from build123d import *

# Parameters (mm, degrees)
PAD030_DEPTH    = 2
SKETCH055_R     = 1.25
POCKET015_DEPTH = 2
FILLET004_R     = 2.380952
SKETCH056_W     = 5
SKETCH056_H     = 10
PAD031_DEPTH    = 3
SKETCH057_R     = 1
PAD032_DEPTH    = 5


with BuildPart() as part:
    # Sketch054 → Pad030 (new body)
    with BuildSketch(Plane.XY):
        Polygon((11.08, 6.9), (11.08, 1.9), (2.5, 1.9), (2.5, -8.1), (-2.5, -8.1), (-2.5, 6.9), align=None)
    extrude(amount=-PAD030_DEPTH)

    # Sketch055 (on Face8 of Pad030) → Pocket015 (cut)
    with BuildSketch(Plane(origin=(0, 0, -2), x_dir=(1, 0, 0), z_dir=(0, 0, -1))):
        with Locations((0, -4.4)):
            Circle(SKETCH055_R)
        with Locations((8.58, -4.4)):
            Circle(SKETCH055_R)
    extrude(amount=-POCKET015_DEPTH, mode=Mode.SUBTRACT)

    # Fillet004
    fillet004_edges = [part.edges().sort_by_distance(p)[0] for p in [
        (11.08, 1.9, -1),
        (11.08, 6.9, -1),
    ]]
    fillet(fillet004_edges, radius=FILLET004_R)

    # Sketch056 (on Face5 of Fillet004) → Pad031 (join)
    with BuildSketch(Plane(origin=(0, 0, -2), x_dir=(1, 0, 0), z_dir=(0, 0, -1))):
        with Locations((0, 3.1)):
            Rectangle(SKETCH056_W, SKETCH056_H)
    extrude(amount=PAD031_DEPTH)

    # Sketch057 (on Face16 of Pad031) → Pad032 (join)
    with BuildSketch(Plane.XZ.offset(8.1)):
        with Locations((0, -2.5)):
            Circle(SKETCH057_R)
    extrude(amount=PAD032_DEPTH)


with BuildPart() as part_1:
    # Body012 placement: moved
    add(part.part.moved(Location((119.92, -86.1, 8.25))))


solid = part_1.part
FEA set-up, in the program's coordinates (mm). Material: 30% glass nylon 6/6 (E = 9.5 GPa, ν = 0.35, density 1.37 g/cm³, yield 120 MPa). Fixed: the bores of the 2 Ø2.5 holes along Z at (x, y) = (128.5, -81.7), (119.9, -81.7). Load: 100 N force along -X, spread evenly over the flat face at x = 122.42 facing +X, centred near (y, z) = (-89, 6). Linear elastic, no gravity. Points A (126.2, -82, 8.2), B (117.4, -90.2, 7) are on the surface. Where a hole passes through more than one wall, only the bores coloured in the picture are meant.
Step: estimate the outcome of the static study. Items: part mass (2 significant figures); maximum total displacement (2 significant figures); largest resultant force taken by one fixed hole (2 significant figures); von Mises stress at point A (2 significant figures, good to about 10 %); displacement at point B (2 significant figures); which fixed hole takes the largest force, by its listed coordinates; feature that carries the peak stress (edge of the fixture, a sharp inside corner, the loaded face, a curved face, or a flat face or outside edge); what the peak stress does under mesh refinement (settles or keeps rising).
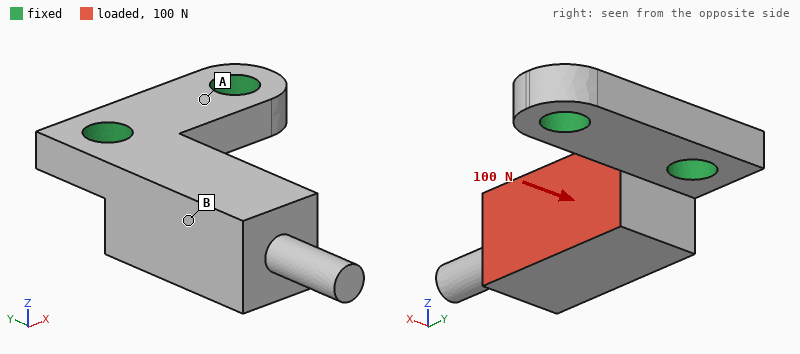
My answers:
0.52 g
0.19 mm
74 N
16 MPa
0.084 mm
(119.9, -81.7)
a sharp inside corner
keeps rising
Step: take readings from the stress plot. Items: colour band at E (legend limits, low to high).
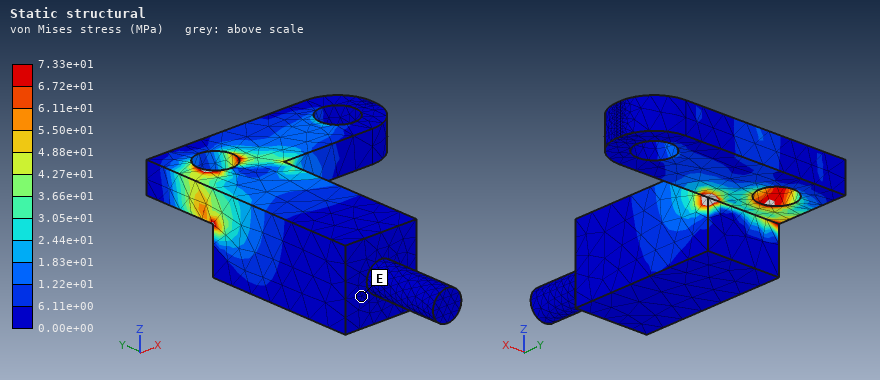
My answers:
0.00e+00 to 6.11e+00 MPa
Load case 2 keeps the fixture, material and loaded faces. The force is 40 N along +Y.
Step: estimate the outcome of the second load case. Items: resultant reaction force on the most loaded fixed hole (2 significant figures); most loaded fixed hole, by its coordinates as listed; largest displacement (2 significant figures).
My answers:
33 N
(119.9, -81.7)
78 µm
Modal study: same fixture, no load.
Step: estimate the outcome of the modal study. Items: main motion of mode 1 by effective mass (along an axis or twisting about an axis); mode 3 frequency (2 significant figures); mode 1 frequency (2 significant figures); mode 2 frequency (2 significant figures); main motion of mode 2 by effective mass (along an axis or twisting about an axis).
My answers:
along Z
18 kHz
4100 Hz
7900 Hz
along X
